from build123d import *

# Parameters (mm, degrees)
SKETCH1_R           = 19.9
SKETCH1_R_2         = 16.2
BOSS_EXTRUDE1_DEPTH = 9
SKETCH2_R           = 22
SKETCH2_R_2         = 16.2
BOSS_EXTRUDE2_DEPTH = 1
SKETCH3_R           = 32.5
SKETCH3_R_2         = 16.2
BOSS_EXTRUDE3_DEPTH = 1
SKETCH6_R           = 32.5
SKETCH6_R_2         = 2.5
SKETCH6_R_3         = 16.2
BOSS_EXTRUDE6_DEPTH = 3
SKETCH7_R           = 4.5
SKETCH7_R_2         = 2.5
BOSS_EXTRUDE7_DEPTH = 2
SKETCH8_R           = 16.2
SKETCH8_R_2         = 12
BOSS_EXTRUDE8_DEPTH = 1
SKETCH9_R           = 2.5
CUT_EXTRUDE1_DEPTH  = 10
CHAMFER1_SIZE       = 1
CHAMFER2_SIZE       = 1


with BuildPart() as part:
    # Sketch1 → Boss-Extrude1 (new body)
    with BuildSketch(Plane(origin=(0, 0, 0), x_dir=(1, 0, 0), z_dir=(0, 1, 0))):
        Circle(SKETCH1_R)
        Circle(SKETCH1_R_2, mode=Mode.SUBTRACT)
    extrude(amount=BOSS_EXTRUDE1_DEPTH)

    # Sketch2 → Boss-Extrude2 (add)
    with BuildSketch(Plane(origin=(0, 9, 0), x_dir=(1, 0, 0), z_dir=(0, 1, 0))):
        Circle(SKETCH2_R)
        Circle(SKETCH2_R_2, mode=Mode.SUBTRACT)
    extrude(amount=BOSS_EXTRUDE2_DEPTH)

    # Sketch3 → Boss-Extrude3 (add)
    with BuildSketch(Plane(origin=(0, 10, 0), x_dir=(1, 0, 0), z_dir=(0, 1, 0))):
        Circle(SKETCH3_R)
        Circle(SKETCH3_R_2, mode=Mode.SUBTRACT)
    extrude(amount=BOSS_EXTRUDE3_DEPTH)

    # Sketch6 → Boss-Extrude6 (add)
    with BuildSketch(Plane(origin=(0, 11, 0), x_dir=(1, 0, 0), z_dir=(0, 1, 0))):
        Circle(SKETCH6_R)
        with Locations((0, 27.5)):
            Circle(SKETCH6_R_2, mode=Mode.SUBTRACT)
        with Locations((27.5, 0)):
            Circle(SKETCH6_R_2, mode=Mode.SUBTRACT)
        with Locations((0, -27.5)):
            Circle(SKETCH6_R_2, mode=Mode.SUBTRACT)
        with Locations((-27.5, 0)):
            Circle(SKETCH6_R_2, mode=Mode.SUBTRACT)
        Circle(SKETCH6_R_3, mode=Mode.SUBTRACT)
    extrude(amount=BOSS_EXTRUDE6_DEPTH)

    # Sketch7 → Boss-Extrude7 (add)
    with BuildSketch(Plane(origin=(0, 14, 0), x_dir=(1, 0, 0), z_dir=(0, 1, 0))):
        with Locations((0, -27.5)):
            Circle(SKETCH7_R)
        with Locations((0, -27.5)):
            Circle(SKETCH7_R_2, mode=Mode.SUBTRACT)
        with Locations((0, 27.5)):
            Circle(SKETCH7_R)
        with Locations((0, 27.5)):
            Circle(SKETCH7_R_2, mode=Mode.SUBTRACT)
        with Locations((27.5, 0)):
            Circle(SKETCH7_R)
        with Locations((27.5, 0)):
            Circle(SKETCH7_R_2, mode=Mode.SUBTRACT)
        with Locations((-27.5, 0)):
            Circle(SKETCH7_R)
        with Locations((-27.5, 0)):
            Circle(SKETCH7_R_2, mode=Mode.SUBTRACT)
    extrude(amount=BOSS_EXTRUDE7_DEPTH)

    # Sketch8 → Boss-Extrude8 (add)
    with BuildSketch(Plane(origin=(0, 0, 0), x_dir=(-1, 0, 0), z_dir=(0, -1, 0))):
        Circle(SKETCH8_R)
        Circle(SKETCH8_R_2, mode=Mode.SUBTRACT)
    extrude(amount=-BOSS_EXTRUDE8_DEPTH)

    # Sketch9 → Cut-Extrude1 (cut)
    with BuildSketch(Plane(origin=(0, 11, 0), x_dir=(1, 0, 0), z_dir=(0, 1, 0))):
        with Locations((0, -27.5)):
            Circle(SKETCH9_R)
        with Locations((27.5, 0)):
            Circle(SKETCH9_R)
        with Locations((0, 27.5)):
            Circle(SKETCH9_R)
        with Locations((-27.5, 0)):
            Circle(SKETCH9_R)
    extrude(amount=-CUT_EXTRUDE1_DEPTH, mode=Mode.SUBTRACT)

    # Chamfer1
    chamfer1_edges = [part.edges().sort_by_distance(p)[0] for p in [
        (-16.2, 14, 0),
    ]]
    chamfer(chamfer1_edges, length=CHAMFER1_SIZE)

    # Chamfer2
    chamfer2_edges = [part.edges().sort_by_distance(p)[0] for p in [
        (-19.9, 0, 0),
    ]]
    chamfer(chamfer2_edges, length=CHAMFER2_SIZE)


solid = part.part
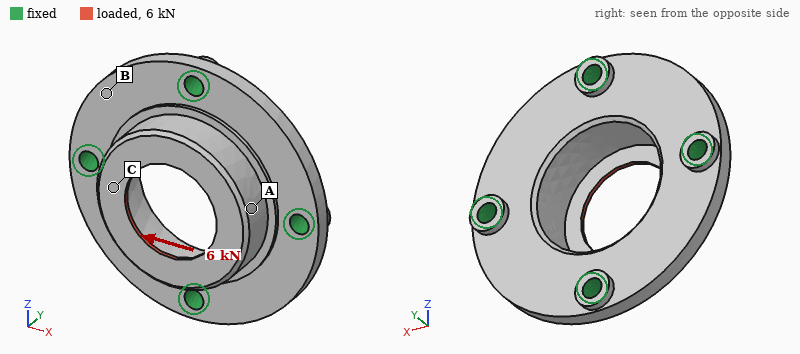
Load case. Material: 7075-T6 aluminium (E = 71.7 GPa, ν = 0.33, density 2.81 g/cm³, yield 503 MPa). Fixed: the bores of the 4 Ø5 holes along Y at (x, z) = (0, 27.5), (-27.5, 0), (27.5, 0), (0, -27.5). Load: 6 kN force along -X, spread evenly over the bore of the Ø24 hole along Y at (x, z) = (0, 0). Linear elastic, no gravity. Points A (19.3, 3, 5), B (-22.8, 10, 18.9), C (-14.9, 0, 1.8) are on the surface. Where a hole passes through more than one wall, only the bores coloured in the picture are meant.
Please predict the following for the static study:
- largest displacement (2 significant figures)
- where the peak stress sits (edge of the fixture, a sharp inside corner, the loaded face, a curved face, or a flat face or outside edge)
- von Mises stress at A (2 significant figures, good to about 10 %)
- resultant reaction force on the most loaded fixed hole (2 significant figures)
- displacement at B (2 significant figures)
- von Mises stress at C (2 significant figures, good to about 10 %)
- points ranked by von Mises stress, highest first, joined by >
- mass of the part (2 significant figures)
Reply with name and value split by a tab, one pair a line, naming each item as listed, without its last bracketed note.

largest displacement	49 µm
where the peak stress sits	a sharp inside corner
von Mises stress at A	52 MPa
resultant reaction force on the most loaded fixed hole	2.1 kN
displacement at B	14 µm
von Mises stress at C	130 MPa
points ranked by von Mises stress, highest first, joined by >	C > A > B
mass of the part	41 g
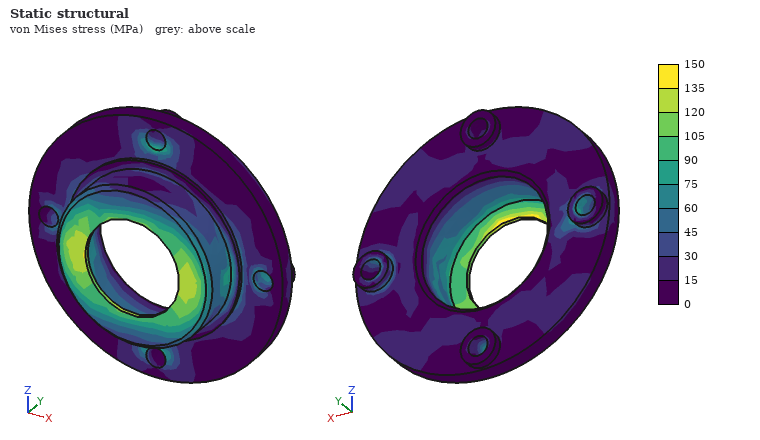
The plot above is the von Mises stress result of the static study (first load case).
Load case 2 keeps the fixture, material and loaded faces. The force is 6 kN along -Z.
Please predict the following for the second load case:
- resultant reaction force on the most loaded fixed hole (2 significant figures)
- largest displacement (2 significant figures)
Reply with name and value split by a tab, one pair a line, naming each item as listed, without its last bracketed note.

resultant reaction force on the most loaded fixed hole	2.1 kN
largest displacement	48 µm
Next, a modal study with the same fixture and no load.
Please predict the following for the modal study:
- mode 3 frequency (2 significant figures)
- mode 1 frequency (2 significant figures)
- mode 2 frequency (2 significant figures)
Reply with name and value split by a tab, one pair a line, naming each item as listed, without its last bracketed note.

mode 3 frequency	15 kHz
mode 1 frequency	14 kHz
mode 2 frequency	15 kHz
